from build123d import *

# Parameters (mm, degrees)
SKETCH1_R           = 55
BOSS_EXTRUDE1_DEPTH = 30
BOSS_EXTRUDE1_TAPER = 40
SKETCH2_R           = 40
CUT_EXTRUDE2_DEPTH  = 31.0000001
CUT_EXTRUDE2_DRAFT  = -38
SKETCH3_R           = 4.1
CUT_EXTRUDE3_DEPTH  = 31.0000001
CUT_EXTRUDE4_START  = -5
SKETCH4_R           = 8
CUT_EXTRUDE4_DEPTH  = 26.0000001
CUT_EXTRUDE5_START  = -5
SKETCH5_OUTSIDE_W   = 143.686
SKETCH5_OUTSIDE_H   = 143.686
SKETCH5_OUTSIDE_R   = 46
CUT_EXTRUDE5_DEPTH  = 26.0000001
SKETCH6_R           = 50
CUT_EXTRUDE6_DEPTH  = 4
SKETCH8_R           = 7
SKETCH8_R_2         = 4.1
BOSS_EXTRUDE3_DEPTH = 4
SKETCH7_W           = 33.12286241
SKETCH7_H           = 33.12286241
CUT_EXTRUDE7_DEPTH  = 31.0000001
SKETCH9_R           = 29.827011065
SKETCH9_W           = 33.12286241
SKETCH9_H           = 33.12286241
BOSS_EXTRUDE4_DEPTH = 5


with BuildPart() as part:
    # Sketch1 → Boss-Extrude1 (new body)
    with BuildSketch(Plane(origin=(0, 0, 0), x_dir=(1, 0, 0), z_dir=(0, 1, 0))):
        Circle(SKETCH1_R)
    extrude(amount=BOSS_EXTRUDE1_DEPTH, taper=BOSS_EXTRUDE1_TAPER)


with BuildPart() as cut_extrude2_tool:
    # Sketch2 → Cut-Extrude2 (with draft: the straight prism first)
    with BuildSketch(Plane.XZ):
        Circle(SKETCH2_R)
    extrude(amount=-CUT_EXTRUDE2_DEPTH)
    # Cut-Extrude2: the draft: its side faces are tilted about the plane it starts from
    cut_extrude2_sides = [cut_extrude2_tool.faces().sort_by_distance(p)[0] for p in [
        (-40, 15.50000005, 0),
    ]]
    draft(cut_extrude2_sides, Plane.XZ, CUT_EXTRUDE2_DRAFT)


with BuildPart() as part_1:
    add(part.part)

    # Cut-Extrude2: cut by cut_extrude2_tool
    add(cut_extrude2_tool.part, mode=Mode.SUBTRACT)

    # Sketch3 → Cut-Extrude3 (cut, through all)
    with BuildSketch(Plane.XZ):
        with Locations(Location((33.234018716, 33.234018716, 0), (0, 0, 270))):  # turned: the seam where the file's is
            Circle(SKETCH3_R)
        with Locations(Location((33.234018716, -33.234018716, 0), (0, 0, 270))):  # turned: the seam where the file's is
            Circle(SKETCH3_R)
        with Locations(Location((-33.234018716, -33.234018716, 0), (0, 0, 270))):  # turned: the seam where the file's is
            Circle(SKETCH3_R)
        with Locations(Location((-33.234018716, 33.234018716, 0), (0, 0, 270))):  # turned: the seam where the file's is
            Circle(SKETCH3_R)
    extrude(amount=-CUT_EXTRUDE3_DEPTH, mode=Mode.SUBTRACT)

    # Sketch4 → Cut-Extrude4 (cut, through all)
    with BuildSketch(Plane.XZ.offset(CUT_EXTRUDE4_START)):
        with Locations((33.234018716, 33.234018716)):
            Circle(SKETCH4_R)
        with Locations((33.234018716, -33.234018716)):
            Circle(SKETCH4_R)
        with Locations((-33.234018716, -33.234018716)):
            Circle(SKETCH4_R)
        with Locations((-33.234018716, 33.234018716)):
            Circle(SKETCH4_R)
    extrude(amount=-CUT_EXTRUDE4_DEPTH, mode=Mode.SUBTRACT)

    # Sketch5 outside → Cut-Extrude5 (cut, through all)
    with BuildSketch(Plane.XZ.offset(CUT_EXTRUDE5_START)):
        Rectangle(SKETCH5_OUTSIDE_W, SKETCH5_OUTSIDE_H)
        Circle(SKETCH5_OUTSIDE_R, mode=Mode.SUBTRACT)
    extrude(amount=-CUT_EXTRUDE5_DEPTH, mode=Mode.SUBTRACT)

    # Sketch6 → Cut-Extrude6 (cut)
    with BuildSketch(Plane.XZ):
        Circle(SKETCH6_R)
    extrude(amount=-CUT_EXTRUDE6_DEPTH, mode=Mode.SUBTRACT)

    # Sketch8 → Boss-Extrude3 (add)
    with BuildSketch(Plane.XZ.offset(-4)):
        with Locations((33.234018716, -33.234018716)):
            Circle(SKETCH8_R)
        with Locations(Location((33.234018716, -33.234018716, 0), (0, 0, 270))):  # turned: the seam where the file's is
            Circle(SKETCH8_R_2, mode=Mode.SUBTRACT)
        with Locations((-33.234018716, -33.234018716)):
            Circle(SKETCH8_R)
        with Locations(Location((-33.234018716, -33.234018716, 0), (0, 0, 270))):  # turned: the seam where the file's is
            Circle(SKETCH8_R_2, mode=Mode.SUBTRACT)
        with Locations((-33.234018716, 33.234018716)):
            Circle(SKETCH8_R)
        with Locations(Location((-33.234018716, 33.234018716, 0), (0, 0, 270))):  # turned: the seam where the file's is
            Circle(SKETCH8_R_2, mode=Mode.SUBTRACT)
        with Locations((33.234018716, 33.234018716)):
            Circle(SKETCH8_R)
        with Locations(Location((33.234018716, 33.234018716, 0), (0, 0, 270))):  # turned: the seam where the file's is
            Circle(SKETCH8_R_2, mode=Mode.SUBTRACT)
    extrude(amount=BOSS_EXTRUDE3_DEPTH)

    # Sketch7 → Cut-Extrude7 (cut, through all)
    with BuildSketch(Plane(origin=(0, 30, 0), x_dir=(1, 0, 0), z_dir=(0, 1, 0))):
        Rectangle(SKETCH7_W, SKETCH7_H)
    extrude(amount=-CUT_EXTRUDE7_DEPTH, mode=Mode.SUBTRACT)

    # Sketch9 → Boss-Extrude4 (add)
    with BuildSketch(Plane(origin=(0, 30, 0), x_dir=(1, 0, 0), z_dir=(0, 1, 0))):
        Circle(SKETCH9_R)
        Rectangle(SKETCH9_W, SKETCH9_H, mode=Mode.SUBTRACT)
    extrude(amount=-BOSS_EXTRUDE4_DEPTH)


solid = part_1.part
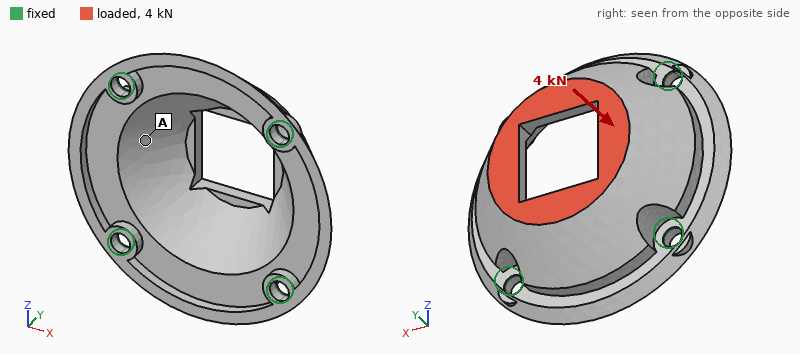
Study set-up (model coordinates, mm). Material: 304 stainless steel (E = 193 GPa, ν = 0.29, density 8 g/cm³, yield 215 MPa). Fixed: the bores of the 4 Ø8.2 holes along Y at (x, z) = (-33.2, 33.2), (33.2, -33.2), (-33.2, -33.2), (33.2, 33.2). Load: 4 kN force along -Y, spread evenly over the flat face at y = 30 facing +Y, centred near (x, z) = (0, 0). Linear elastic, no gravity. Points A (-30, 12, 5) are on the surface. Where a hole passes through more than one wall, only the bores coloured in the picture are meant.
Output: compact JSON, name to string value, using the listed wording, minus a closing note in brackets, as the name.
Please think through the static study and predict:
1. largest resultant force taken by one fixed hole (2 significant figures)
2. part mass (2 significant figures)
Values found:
{"largest resultant force taken by one fixed hole": "1.3 kN", "part mass": "610 g"}
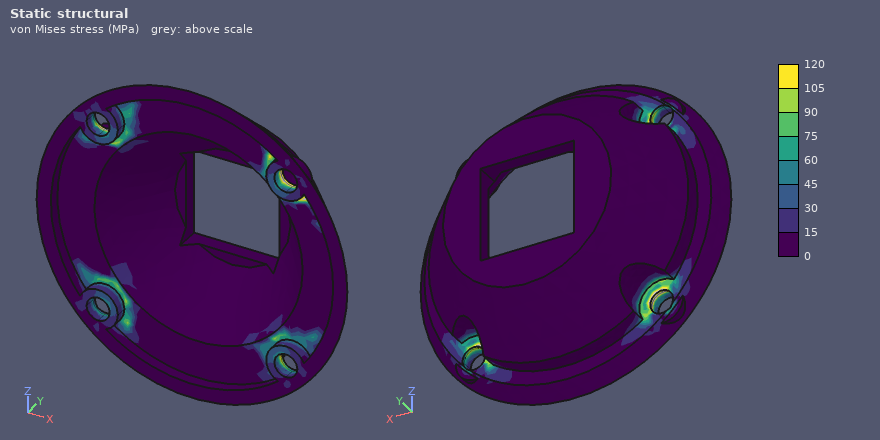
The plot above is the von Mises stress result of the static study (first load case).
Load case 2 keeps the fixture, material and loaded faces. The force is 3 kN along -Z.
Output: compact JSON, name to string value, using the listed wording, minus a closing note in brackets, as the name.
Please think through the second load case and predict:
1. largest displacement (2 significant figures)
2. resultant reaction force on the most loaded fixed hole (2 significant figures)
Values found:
{"largest displacement": "7.6 µm", "resultant reaction force on the most loaded fixed hole": "980 N"}
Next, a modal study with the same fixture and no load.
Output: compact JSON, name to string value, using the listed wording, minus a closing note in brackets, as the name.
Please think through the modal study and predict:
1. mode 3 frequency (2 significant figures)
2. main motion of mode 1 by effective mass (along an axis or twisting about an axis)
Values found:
{"mode 3 frequency": "6100 Hz", "main motion of mode 1 by effective mass": "along Y"}
